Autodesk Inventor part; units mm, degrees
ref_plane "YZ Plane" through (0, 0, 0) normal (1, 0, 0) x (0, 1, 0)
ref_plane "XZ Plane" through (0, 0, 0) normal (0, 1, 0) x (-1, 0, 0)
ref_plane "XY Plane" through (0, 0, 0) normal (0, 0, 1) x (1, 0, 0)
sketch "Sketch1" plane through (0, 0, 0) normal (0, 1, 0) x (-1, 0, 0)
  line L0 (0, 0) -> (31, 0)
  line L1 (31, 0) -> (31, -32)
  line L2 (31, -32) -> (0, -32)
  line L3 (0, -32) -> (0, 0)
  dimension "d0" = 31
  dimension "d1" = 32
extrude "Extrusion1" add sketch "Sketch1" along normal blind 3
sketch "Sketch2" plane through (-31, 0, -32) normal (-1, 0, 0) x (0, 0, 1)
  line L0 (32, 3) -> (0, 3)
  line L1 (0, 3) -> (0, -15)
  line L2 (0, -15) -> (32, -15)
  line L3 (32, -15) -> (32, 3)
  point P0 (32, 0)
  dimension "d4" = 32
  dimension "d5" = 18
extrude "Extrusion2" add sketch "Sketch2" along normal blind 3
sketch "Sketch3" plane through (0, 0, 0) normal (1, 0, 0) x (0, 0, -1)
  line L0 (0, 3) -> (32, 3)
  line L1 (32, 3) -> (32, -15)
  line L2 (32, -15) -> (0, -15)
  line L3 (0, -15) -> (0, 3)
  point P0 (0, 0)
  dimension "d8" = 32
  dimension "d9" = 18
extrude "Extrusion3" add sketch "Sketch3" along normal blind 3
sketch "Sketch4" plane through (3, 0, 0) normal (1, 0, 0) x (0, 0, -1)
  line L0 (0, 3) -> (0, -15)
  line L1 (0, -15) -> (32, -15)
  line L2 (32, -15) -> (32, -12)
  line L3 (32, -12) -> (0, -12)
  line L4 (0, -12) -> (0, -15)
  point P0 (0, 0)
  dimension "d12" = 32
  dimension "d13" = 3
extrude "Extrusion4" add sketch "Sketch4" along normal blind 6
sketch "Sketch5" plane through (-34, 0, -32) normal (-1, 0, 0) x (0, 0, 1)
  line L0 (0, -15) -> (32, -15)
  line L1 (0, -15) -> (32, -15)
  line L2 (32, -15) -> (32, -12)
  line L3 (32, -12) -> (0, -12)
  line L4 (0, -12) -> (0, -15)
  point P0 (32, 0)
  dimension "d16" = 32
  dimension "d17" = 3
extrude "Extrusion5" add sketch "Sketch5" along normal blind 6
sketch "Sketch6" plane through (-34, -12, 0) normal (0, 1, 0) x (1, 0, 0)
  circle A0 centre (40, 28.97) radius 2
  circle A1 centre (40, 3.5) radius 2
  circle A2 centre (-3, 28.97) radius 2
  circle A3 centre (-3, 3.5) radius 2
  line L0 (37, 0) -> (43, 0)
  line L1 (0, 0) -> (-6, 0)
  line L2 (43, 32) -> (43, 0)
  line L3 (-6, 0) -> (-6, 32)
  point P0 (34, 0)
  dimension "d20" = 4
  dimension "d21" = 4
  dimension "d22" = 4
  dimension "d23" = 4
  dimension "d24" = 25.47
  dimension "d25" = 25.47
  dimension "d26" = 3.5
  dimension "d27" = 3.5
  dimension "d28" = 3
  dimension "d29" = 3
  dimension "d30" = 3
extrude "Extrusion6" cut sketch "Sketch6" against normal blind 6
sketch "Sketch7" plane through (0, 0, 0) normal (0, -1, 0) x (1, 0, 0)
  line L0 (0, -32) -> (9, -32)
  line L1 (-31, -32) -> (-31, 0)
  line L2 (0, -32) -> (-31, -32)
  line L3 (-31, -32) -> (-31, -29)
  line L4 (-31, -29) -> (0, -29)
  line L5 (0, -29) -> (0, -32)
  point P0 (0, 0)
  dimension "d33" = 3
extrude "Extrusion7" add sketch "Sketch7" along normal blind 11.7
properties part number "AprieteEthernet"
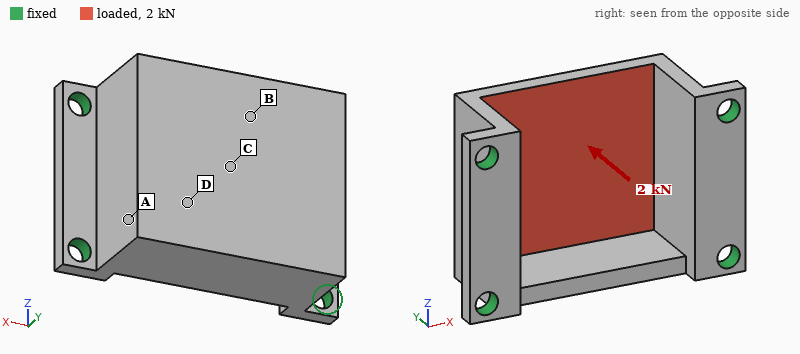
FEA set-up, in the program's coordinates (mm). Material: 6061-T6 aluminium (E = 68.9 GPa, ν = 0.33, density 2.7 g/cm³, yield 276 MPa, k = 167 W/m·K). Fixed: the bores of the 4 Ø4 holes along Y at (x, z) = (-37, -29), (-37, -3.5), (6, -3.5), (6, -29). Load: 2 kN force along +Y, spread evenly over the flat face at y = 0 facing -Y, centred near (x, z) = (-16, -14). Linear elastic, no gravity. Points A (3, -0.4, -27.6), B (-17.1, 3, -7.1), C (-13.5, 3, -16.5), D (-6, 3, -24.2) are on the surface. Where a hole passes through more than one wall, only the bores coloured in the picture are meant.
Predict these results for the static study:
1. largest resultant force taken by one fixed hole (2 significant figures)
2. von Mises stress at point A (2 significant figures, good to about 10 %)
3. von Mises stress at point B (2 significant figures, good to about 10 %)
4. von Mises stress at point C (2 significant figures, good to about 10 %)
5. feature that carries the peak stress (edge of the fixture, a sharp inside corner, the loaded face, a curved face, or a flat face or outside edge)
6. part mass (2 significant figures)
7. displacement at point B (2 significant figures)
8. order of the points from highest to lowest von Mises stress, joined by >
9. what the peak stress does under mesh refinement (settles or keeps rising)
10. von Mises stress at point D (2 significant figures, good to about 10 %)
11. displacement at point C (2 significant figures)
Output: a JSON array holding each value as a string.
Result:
["630 N", "17 MPa", "75 MPa", "57 MPa", "edge of the fixture", "23 g", "70 µm", "B > C > D > A", "keeps rising", "37 MPa", "51 µm"]
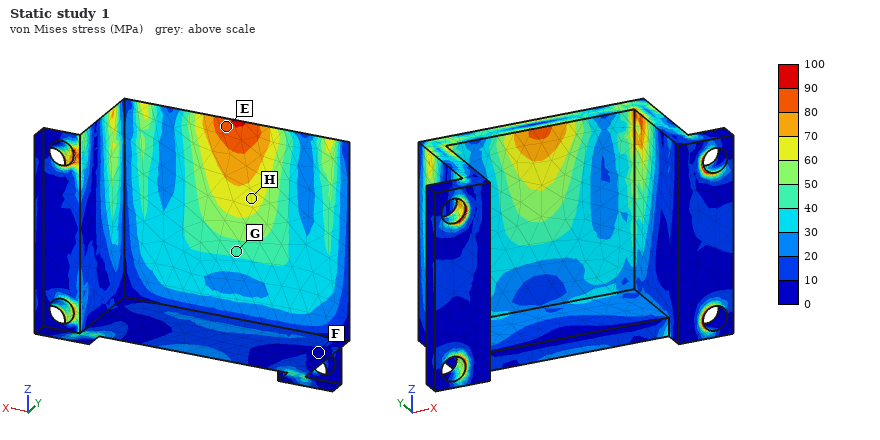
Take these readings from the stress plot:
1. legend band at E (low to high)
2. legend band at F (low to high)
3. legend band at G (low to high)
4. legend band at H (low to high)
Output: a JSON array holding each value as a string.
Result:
["80 to 90 MPa", "0 to 10 MPa", "40 to 50 MPa", "60 to 70 MPa"]
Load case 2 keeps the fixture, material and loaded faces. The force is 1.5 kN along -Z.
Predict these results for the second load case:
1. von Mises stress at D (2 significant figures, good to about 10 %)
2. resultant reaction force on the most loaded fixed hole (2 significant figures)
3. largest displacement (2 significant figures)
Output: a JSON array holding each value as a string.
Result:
["9.1 MPa", "560 N", "17 µm"]
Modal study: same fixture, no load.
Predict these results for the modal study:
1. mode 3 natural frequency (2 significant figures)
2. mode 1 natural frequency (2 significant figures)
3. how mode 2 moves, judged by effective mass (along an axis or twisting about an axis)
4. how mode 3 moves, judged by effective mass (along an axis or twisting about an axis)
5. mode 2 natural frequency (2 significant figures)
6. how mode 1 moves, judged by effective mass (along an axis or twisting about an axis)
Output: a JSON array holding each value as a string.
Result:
["14 kHz", "9700 Hz", "along Y", "along Z", "11 kHz", "along X"]
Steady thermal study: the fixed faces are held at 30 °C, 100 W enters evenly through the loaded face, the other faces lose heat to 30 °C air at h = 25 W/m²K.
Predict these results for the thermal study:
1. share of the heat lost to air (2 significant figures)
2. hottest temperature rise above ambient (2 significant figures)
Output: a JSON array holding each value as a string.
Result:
["5.1 %", "79 K"]
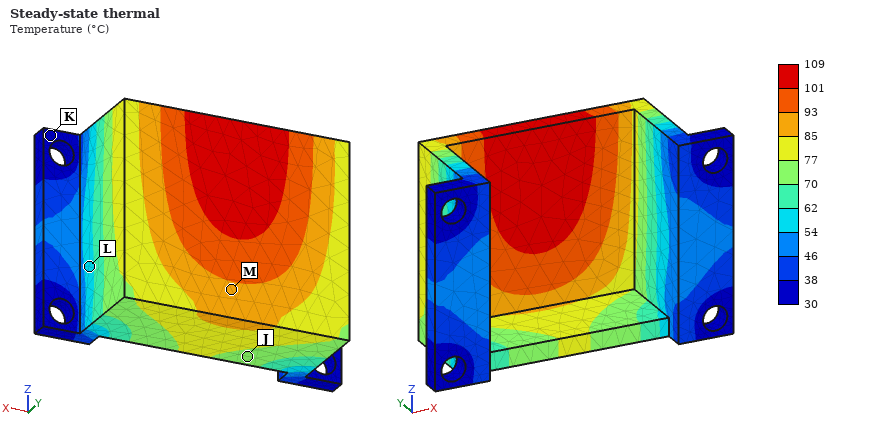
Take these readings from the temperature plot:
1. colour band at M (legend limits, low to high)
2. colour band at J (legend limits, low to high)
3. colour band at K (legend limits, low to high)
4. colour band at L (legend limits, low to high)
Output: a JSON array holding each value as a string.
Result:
["85 to 93 °C", "70 to 77 °C", "30 to 38 °C", "54 to 62 °C"]
